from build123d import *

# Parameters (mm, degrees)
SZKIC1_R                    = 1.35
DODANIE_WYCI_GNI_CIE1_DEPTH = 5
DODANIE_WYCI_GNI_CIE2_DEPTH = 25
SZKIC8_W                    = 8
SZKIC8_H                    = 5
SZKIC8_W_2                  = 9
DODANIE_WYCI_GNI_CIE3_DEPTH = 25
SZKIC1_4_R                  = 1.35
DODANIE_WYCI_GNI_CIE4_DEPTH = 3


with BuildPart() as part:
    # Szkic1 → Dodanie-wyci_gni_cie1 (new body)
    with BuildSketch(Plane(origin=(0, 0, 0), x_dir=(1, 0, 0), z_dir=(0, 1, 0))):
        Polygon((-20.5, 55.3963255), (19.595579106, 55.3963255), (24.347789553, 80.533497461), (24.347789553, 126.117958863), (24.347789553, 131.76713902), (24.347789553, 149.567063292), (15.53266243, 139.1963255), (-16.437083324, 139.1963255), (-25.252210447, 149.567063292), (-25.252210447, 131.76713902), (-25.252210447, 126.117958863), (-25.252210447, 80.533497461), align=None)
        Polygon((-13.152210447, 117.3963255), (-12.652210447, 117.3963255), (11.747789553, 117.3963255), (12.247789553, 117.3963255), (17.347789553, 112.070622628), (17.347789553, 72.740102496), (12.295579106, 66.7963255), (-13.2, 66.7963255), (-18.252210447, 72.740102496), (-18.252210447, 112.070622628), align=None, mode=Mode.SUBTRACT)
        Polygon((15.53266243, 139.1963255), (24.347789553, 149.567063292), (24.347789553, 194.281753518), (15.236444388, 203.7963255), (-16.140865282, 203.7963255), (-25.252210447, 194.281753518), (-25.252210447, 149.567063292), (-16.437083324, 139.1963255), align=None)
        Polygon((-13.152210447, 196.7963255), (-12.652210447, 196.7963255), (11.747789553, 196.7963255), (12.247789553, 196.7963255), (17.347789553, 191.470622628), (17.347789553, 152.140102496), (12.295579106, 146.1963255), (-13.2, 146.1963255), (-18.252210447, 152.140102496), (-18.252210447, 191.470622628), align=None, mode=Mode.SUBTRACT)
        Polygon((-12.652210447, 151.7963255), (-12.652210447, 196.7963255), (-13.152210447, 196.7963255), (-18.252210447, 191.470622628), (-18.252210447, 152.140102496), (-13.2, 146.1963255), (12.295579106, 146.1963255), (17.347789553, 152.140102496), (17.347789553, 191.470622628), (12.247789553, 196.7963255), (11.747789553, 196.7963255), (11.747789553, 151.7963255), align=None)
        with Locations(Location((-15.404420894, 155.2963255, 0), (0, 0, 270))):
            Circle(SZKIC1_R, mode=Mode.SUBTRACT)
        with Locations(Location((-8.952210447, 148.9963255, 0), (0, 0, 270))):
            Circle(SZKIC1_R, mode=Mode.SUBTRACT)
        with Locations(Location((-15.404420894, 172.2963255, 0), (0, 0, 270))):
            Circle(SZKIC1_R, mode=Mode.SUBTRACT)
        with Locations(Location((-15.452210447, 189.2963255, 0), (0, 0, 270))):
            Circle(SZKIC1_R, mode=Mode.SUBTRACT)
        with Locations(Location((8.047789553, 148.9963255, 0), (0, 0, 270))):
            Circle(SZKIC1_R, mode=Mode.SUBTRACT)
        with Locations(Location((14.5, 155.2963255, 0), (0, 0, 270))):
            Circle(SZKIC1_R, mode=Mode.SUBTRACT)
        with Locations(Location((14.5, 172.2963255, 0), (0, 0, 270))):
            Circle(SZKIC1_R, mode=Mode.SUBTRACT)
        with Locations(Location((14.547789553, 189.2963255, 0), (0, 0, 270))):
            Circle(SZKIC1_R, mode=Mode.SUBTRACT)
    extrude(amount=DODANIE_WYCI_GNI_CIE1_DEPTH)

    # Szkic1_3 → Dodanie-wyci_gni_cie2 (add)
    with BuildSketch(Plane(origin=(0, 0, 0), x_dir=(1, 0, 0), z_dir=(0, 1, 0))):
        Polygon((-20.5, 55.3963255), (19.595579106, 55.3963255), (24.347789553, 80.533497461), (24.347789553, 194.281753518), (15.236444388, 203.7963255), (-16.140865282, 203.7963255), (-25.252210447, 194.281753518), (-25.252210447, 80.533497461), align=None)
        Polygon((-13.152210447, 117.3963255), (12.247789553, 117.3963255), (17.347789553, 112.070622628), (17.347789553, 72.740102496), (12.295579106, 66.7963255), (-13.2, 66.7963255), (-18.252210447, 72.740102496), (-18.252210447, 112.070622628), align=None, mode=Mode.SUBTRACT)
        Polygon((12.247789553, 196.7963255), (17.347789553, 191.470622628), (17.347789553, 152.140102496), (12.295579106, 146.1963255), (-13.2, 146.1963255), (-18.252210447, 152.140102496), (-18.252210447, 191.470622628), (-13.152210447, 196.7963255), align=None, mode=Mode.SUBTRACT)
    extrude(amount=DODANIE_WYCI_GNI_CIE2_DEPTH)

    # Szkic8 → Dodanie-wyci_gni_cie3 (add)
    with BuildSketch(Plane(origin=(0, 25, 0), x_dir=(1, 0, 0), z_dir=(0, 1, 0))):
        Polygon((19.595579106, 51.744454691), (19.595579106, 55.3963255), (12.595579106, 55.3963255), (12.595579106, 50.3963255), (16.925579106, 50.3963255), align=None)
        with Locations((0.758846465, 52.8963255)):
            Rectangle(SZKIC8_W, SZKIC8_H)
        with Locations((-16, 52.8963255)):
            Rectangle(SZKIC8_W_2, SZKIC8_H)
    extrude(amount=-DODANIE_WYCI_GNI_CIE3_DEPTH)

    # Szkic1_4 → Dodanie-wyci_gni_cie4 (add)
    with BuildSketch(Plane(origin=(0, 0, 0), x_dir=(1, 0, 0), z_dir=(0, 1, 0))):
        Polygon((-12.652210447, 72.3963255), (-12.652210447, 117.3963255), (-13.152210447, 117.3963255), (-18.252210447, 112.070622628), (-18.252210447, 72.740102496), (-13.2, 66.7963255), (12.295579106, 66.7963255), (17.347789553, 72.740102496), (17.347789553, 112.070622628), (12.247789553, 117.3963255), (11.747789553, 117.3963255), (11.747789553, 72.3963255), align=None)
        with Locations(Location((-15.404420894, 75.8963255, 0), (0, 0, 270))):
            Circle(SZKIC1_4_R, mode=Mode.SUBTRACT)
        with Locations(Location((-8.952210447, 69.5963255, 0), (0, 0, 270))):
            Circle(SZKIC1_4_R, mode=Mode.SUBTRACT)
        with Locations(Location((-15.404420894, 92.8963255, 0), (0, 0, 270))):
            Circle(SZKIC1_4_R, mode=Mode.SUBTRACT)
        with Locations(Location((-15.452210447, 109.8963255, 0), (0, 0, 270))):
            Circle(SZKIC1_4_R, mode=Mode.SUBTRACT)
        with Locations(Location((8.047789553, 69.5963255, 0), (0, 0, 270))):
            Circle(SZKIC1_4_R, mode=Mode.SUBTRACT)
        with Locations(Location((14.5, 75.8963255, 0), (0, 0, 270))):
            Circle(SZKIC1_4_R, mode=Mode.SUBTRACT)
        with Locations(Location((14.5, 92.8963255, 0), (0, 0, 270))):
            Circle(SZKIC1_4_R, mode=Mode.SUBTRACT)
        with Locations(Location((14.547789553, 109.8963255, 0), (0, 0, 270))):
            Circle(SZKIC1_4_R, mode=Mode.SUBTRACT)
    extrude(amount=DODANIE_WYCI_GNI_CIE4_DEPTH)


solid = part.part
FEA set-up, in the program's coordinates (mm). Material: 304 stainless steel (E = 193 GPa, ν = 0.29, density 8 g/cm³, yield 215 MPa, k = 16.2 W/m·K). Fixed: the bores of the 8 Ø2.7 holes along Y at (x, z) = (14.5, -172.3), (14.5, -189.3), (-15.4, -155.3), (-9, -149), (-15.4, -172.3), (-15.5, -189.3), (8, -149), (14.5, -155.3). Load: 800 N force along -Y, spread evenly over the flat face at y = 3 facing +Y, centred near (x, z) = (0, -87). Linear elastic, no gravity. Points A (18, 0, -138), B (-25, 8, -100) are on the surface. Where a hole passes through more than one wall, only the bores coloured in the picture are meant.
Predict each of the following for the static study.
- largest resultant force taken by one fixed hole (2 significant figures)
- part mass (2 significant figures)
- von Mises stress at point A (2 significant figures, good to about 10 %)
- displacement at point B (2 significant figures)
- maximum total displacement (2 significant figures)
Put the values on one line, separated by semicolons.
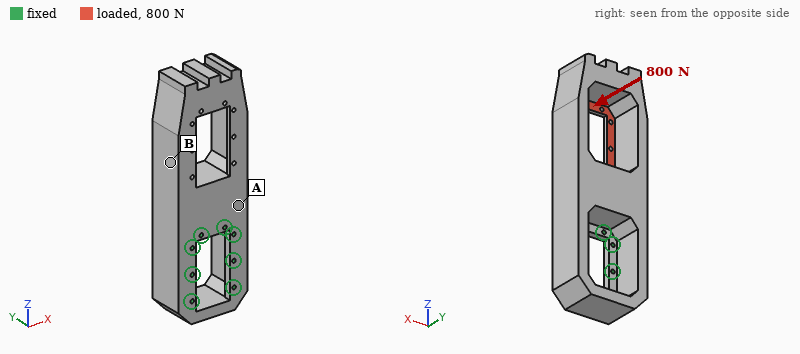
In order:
1.0 kN; 800 g; 9.7 MPa; 17 µm; 41 µm
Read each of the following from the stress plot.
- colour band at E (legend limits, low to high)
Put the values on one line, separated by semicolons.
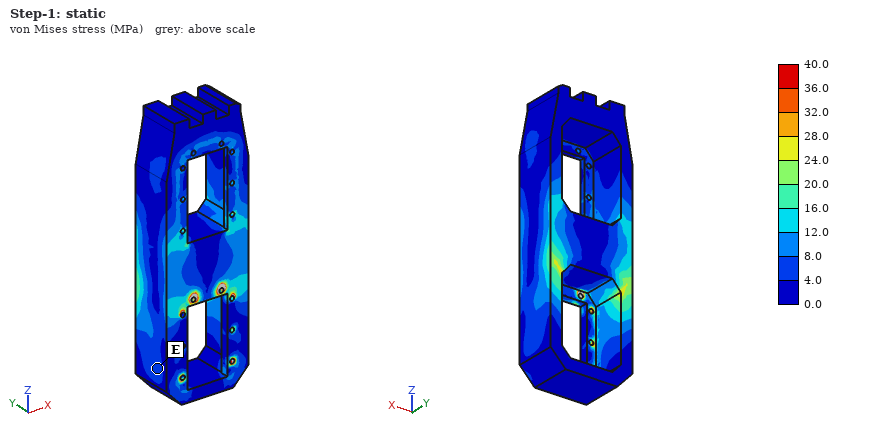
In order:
4.0 to 8.0 MPa
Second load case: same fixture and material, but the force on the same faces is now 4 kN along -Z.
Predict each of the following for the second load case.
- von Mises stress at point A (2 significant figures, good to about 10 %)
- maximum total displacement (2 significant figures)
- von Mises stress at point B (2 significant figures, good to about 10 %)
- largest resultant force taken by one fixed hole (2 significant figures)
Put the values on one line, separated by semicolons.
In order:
14 MPa; 26 µm; 9.0 MPa; 1.0 kN
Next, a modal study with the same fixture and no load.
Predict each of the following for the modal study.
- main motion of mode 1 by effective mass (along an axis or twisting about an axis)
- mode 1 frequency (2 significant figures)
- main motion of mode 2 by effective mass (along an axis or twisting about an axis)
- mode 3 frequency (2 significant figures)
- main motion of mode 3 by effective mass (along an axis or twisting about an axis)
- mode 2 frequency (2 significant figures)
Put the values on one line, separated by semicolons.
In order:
along Y; 1400 Hz; along X; 3500 Hz; twisting about Z; 1700 Hz
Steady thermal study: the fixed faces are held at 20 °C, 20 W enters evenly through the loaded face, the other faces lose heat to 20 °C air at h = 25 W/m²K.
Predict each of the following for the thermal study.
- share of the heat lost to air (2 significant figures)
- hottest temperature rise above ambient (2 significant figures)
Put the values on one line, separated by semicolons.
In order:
73 %; 68 K
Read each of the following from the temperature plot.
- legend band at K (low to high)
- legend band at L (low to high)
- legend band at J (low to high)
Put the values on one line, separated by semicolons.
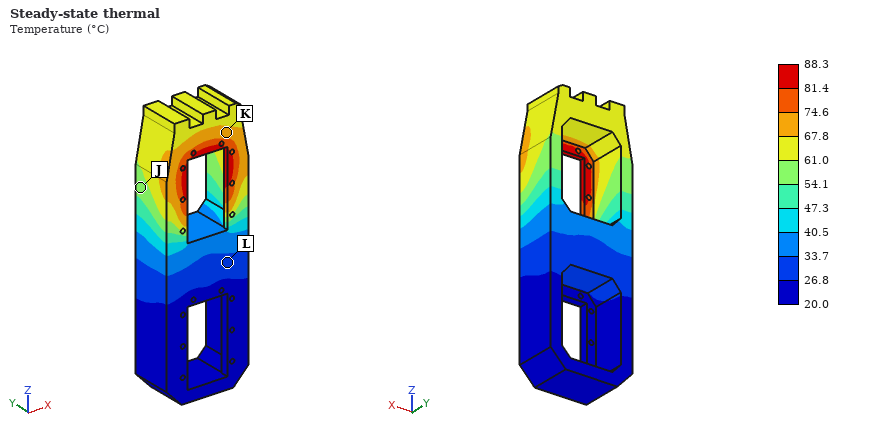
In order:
67.8 to 74.6 °C; 26.8 to 33.7 °C; 54.1 to 61.0 °C
